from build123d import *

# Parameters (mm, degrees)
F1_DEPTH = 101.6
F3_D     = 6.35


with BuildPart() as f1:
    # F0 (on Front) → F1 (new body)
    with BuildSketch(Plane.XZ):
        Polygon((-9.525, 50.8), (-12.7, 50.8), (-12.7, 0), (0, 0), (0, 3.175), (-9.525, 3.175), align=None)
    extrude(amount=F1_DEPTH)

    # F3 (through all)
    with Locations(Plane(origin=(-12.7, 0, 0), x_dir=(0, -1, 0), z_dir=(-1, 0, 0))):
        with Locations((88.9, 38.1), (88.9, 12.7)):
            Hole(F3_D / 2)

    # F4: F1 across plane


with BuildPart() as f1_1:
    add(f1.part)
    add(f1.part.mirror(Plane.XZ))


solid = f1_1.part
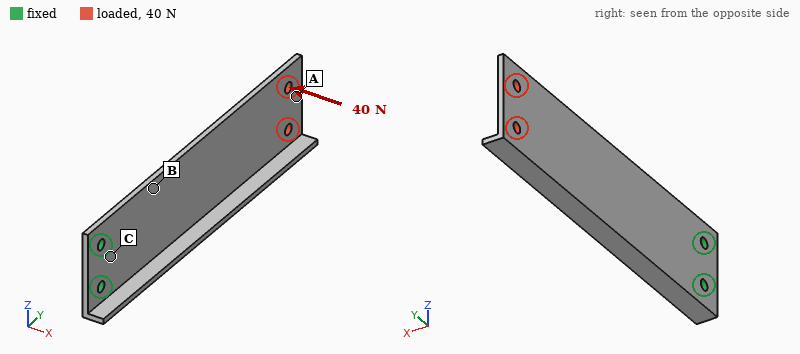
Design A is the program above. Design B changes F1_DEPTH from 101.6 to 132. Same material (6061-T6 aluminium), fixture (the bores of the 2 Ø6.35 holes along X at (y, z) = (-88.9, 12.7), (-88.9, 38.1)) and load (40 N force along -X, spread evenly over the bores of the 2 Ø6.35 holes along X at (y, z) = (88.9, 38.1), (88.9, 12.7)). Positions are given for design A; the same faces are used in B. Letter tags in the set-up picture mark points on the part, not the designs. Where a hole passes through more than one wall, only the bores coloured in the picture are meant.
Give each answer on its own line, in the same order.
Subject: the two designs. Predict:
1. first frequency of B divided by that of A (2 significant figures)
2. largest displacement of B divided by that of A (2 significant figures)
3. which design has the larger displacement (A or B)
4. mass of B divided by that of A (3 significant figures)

0.79
1.1
B
1.30
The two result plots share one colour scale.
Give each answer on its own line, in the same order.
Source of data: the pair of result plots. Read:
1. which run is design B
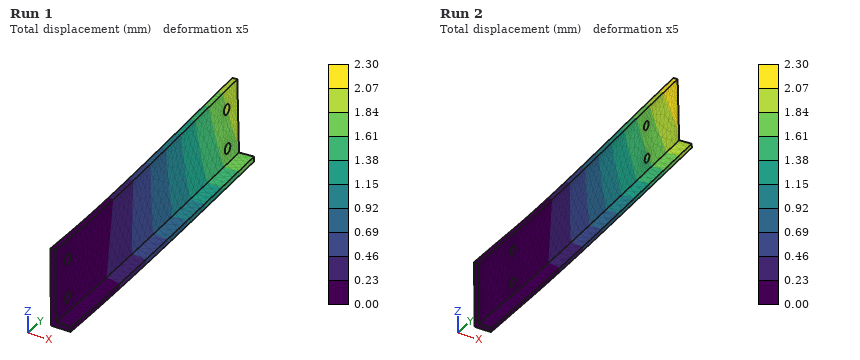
Run 2
